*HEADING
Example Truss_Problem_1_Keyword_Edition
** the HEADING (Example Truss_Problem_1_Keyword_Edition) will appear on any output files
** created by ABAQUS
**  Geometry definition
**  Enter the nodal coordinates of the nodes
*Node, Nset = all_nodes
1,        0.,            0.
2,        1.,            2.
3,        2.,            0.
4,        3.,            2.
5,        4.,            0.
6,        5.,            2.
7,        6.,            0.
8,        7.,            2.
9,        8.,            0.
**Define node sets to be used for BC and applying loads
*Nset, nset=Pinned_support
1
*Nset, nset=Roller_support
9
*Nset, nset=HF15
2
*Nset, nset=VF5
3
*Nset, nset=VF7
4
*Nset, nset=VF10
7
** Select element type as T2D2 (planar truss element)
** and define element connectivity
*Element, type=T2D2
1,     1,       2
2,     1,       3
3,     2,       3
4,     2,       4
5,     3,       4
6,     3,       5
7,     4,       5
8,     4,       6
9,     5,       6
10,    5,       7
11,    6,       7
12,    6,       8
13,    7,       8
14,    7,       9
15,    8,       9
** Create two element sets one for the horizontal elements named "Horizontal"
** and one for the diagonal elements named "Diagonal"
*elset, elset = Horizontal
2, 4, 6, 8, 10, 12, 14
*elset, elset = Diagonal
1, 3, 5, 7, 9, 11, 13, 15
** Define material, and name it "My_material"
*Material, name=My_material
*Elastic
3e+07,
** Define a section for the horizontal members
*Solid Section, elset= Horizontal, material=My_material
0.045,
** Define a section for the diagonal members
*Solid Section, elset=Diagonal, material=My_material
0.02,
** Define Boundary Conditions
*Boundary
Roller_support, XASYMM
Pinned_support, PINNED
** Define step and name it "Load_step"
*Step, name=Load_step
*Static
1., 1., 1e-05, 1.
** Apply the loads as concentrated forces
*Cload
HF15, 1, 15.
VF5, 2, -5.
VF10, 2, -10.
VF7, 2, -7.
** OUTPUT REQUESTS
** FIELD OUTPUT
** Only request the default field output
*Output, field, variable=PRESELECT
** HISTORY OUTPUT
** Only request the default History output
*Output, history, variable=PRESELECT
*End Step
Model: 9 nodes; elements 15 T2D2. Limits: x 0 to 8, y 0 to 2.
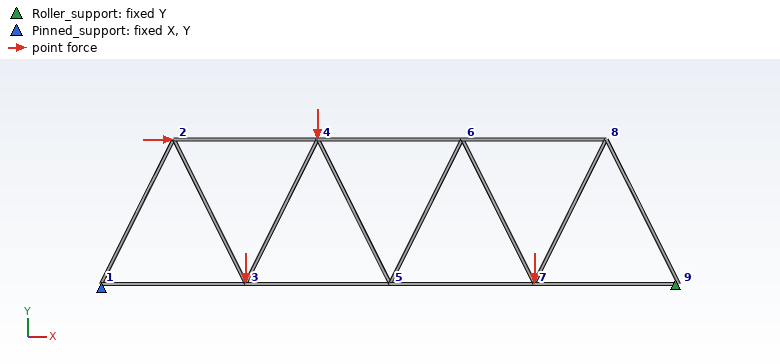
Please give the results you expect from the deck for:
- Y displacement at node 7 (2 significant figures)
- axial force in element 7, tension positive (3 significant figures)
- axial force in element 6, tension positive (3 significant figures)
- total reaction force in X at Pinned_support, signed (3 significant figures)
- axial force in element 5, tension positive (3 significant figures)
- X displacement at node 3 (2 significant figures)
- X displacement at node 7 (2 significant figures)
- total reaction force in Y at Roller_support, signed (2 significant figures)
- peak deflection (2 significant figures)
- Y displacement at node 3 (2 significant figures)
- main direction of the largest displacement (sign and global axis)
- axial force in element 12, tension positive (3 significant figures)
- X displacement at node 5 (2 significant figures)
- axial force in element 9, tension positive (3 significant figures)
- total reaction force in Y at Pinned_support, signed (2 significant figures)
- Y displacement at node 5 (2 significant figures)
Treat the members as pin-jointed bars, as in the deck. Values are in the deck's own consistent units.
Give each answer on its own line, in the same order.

-1.8e-04
-5.73
22.8
-15.0
-2.10
2.7e-05
8.7e-05
15
2.6e-04
-1.9e-04
-Y
-15.1
6.1e-05
5.73
6.9
-2.3e-04
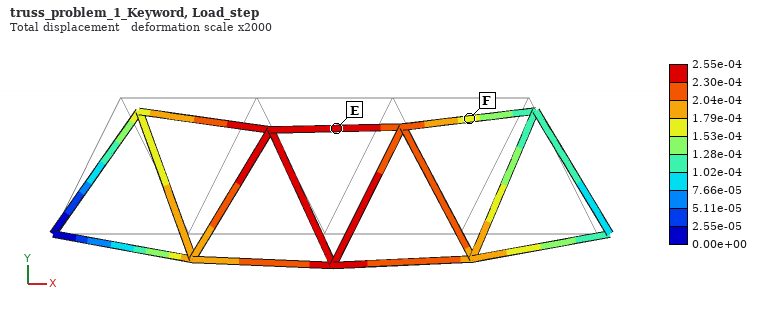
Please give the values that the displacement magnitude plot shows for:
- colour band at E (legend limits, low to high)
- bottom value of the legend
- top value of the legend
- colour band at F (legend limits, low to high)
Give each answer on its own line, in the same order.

2.30e-04 to 2.55e-04
0.00e+00
2.55e-04
1.53e-04 to 1.79e-04
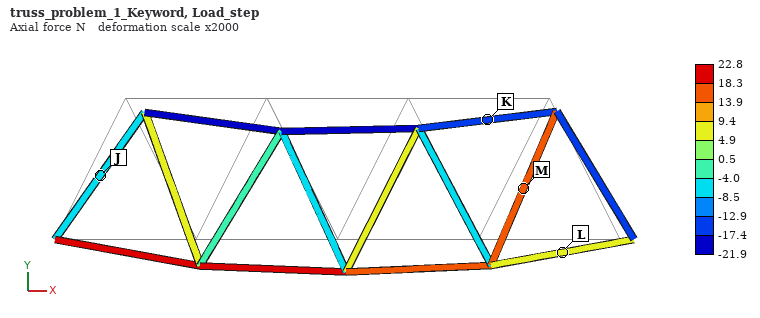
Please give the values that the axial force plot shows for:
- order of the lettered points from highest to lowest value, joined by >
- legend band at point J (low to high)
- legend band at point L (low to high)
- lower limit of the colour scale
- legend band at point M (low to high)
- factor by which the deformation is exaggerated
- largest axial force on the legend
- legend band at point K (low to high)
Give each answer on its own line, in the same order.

M > L > J > K
-8.5 to -4.0
4.9 to 9.4
-21.9
13.9 to 18.3
2000
22.8
-17.4 to -12.9
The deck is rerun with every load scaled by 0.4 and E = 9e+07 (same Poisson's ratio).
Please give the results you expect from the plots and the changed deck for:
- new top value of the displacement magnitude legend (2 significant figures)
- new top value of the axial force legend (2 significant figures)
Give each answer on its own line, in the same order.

3.4e-05
9.1
